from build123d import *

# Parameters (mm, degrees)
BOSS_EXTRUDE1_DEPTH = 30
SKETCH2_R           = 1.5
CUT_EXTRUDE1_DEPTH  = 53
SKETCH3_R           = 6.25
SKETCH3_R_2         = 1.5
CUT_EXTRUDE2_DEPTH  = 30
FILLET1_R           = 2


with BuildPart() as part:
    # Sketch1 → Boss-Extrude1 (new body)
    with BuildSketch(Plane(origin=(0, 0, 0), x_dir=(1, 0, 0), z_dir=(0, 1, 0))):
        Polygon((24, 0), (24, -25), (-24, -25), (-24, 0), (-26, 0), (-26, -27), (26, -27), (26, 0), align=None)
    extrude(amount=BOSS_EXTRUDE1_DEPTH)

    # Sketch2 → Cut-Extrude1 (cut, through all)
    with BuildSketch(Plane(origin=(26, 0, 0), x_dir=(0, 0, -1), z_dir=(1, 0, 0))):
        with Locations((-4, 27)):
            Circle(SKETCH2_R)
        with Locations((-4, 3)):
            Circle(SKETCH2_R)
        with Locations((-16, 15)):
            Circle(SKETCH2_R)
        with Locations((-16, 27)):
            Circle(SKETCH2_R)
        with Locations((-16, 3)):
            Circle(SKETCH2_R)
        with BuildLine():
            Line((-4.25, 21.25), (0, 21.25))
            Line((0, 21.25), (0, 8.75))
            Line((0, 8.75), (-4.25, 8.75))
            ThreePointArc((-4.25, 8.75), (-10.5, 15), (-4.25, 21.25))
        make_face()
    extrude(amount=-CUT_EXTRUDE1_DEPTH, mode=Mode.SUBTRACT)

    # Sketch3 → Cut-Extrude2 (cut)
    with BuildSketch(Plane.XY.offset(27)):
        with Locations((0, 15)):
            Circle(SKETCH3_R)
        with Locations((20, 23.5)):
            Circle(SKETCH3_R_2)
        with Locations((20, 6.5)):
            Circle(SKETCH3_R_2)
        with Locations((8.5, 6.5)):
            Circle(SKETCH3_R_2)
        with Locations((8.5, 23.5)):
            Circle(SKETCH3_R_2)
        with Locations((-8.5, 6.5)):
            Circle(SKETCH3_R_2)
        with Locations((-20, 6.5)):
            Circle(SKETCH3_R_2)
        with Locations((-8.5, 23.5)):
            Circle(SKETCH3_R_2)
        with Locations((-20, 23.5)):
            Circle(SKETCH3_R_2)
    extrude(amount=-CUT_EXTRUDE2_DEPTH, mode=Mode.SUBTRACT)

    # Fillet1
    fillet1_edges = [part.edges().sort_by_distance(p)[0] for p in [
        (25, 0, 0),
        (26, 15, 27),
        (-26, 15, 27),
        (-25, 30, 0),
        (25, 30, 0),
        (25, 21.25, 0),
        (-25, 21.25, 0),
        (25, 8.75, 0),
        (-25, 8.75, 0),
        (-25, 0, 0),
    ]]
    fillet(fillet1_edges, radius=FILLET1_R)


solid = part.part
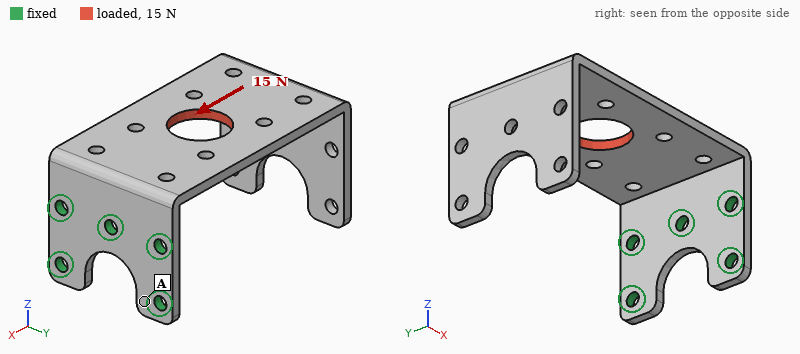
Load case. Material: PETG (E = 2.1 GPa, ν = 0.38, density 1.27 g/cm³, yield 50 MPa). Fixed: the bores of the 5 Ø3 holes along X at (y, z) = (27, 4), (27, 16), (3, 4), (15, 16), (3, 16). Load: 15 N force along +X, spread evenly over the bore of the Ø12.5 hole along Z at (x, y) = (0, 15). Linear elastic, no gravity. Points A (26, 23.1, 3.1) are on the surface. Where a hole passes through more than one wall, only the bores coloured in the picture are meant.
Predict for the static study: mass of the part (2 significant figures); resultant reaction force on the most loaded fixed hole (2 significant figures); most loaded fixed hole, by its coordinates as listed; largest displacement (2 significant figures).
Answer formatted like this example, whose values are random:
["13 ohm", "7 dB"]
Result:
["6.5 g", "6.2 N", "(15, 16)", "0.78 mm"]
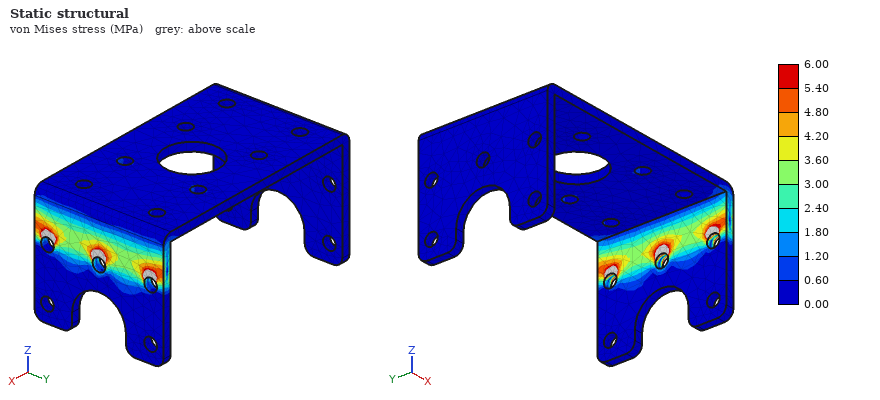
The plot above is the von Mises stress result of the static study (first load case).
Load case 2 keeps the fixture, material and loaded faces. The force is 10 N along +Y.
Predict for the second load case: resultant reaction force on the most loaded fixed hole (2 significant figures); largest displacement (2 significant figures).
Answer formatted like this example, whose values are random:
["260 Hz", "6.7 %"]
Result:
["12 N", "0.73 mm"]
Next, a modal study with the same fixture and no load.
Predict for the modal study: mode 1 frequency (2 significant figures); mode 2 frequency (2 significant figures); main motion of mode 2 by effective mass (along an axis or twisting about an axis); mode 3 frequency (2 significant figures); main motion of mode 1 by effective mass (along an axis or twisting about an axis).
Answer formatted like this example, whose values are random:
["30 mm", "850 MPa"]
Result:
["77 Hz", "200 Hz", "along Y", "350 Hz", "along Z"]
